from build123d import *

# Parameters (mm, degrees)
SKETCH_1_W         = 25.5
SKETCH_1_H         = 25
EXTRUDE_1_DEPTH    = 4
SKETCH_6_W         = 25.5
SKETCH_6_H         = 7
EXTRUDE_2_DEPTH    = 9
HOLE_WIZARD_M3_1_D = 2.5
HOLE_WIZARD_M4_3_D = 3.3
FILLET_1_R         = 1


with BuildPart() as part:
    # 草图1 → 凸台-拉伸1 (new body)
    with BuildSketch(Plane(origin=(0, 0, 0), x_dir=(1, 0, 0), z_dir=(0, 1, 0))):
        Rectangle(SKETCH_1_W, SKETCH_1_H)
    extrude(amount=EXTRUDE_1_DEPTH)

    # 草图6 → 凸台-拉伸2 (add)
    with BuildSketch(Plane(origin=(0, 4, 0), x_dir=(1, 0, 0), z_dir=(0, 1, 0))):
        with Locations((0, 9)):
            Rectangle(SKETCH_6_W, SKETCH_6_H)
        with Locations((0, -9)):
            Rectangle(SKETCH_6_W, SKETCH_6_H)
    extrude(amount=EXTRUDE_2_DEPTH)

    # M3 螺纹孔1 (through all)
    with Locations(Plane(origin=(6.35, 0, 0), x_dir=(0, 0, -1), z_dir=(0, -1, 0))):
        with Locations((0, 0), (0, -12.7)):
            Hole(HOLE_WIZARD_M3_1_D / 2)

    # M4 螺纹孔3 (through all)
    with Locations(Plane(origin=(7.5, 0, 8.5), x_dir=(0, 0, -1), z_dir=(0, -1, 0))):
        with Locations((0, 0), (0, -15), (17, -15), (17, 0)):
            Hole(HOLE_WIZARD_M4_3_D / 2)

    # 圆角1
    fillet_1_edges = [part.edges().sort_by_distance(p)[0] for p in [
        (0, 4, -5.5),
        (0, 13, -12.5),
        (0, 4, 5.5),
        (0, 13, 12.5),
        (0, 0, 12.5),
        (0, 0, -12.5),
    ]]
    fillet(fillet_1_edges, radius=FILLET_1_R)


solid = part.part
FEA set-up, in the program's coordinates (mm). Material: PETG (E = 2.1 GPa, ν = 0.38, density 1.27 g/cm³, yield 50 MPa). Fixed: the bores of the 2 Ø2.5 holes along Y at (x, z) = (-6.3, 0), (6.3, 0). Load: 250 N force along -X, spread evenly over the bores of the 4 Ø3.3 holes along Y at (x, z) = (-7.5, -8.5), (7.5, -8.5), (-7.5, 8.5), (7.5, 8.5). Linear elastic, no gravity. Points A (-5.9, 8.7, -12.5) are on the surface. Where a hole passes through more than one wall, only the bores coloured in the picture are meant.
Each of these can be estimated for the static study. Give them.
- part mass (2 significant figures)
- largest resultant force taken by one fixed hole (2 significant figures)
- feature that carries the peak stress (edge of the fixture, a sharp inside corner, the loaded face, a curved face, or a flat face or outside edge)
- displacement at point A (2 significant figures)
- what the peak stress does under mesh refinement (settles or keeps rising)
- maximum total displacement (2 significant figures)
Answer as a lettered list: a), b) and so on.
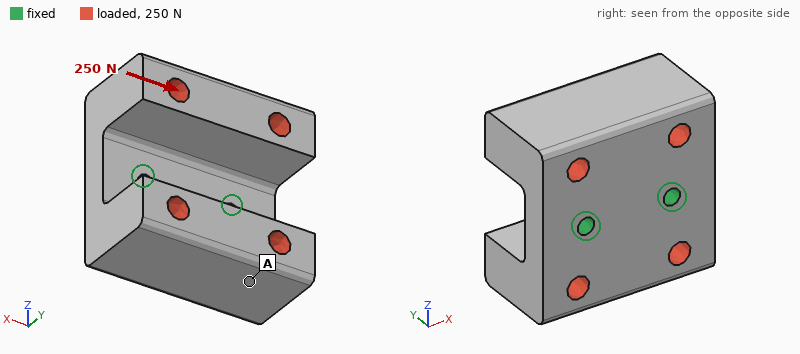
a) 6.7 g
b) 140 N
c) edge of the fixture
d) 40 µm
e) keeps rising
f) 62 µm
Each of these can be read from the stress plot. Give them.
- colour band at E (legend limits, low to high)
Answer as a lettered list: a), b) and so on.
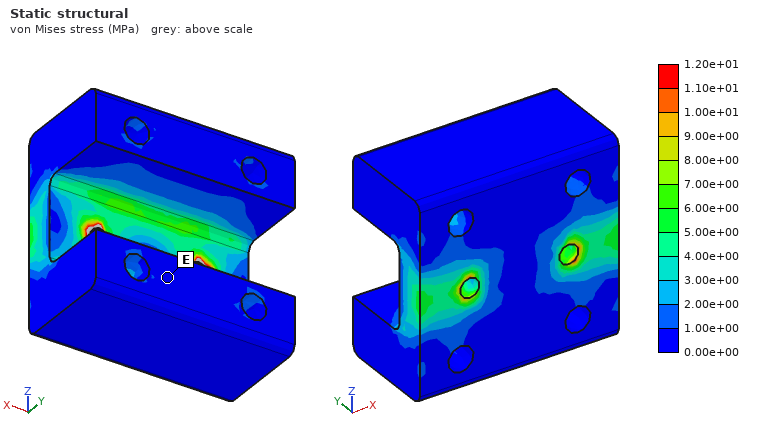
a) 0.00e+00 to 1.00e+00 MPa
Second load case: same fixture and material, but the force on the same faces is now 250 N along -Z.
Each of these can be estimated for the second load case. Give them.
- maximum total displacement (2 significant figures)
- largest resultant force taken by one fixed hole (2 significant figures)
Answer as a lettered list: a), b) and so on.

a) 0.24 mm
b) 130 N
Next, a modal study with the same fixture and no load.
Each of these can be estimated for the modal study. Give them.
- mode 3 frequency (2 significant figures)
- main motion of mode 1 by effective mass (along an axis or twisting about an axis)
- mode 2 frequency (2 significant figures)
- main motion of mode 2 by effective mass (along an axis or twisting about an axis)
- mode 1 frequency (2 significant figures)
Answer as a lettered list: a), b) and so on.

a) 4000 Hz
b) along Z
c) 2500 Hz
d) along Y
e) 2000 Hz
